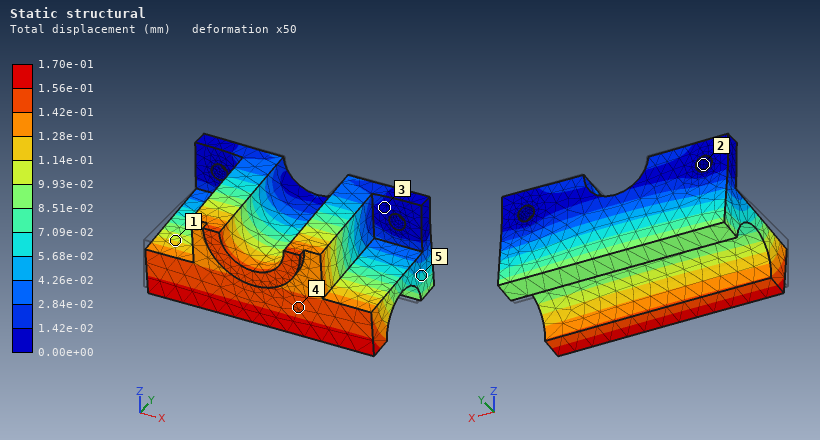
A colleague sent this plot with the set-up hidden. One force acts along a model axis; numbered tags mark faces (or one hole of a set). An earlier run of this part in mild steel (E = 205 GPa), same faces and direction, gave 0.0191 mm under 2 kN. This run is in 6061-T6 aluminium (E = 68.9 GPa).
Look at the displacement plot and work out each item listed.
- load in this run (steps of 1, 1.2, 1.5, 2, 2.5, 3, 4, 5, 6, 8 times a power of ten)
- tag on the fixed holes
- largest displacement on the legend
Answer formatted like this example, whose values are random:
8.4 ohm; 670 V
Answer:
6 kN; 2; 1.70e-01 mm
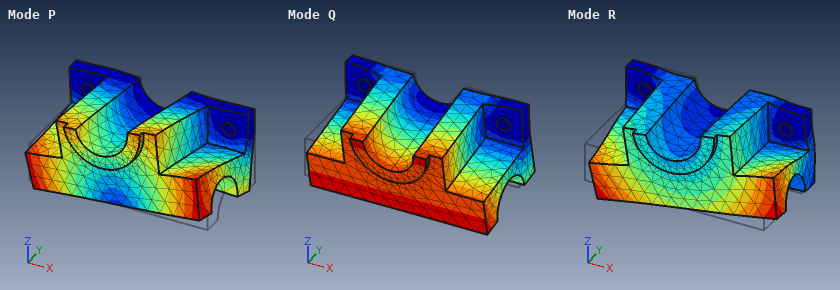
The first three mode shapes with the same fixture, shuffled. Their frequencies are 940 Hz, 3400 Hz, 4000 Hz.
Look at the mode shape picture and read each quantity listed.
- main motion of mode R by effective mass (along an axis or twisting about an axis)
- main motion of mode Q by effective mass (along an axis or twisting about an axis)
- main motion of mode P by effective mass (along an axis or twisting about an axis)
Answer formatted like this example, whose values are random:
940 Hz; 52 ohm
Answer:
along X; along Z; along X
